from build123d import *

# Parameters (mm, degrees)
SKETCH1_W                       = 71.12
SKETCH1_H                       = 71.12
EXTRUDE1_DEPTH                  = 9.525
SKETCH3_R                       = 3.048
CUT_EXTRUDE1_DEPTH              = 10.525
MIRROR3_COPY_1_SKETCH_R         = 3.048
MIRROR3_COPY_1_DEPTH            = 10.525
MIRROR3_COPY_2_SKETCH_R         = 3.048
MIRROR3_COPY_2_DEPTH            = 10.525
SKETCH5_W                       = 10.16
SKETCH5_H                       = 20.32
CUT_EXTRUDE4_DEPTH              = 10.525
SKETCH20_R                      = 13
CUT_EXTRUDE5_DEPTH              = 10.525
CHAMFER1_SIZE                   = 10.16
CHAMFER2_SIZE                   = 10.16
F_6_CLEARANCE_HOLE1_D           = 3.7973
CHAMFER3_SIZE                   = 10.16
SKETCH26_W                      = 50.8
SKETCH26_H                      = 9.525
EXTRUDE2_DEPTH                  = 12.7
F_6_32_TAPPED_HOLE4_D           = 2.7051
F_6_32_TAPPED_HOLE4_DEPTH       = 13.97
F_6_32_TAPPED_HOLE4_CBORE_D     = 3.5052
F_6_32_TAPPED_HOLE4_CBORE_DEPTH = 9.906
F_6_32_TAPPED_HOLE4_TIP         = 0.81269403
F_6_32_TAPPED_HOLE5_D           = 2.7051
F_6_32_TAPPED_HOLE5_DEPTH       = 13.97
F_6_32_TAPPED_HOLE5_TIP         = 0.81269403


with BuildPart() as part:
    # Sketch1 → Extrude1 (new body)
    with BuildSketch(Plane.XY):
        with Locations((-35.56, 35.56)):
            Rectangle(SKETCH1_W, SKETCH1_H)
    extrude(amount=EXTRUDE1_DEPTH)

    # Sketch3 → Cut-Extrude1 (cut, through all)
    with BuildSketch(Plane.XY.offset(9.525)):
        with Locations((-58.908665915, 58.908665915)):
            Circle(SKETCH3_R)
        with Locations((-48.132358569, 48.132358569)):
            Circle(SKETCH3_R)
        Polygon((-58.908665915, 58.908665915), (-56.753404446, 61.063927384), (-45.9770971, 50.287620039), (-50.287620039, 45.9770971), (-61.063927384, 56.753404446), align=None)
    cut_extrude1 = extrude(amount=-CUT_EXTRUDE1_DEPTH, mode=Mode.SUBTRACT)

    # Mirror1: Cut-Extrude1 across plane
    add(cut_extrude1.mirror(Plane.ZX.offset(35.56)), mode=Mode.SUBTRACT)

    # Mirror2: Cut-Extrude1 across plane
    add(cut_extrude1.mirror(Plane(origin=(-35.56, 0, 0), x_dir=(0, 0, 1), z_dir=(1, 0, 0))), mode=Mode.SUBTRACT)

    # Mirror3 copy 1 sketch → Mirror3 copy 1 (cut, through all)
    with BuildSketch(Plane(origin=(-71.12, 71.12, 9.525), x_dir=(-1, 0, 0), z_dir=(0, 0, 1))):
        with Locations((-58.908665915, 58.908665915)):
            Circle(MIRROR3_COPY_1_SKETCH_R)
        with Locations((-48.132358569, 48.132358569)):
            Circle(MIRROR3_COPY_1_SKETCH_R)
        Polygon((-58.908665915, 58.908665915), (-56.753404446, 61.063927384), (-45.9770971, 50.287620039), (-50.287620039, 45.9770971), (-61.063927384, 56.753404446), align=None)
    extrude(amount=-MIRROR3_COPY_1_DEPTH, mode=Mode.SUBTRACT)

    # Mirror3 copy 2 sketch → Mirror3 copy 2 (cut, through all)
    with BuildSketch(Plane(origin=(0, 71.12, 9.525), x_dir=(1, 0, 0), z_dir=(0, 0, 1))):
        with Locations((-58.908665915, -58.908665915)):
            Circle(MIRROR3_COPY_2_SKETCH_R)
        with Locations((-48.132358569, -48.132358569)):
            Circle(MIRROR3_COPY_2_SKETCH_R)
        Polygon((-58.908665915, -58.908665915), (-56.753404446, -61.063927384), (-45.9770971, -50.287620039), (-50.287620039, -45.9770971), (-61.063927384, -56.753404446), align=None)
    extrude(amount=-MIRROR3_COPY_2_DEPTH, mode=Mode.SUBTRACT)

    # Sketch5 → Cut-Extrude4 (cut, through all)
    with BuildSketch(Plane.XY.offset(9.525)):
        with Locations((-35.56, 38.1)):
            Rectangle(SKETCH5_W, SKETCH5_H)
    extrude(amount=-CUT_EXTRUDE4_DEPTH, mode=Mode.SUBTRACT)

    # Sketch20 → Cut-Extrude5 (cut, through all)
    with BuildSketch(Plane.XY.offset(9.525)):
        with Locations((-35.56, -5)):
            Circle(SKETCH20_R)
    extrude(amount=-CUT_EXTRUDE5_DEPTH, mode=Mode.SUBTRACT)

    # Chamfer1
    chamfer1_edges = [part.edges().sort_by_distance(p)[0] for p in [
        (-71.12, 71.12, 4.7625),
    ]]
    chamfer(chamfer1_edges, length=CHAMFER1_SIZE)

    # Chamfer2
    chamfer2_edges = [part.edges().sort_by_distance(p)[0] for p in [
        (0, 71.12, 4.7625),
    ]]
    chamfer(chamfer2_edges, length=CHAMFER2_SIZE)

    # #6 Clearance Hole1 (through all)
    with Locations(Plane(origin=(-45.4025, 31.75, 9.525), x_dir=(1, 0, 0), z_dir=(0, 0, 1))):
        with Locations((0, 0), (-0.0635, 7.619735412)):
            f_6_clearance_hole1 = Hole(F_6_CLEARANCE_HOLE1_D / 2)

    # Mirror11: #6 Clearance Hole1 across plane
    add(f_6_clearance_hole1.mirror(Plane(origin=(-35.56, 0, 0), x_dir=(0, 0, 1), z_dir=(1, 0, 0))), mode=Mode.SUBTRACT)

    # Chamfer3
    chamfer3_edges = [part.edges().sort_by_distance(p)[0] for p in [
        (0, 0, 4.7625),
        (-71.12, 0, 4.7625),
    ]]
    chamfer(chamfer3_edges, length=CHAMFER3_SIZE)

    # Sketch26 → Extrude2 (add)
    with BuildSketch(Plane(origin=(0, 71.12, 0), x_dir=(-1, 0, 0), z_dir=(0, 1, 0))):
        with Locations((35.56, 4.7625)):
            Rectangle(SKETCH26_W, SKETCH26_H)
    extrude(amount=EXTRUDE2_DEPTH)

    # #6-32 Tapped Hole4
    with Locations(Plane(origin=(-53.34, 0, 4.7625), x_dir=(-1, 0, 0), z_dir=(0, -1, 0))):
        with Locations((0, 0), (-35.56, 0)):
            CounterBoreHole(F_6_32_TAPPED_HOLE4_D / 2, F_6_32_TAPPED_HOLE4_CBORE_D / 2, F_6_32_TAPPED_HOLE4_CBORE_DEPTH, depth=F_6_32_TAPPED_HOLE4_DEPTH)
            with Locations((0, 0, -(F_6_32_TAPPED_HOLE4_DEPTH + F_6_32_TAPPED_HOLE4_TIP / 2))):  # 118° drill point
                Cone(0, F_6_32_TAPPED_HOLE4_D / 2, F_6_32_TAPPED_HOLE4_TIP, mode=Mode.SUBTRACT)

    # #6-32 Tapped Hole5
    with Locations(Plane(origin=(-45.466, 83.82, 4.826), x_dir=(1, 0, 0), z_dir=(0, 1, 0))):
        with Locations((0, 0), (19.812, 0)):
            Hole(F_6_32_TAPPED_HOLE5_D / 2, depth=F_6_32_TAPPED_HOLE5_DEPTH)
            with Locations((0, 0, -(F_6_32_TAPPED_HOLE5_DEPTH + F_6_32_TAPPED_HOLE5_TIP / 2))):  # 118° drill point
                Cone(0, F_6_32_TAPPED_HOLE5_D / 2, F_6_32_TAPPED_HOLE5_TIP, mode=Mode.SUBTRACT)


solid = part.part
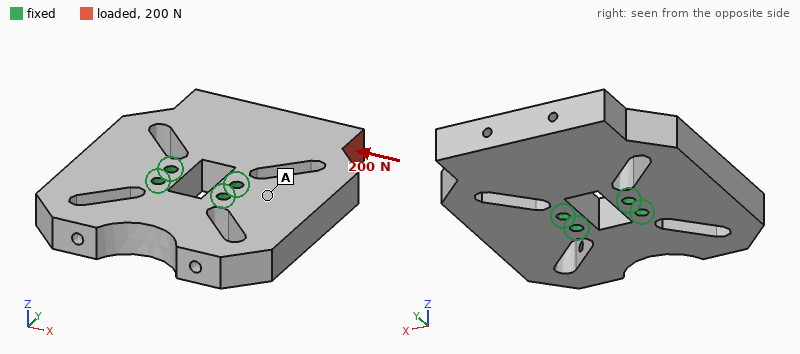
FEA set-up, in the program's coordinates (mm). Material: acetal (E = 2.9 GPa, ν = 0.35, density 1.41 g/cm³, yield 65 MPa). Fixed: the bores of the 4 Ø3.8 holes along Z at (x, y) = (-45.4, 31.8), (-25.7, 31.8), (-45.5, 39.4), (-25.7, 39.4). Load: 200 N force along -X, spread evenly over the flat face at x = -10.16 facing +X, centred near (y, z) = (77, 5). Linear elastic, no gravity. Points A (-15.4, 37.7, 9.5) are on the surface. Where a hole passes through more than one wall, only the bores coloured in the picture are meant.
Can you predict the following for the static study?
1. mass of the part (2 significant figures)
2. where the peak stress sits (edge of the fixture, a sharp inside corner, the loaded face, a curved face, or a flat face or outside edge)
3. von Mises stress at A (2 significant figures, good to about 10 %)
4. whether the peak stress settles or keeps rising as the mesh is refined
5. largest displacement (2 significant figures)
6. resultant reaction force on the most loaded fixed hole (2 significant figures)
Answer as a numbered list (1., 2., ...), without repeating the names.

1. 61 g
2. edge of the fixture
3. 1.0 MPa
4. keeps rising
5. 89 µm
6. 260 N
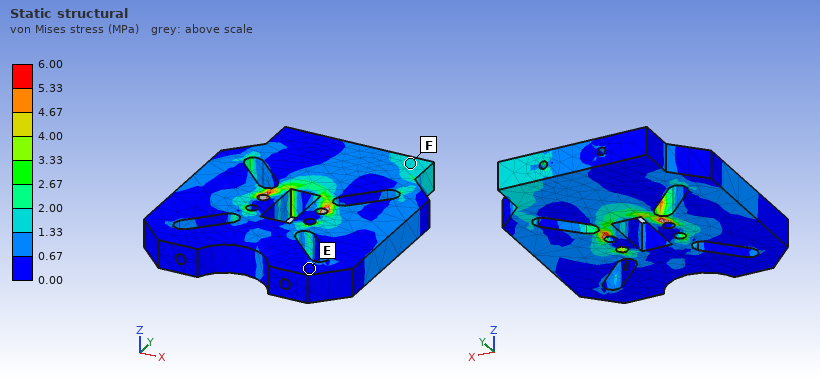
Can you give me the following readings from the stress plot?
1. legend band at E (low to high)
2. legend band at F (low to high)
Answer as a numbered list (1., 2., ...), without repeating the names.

1. 0.00 to 0.67 MPa
2. 1.33 to 2.00 MPa
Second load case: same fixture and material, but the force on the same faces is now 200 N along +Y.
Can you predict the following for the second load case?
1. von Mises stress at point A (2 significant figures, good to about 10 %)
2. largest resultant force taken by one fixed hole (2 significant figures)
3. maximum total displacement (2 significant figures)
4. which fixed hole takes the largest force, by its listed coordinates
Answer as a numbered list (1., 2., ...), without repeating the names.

1. 1.1 MPa
2. 200 N
3. 75 µm
4. (-25.7, 39.4)
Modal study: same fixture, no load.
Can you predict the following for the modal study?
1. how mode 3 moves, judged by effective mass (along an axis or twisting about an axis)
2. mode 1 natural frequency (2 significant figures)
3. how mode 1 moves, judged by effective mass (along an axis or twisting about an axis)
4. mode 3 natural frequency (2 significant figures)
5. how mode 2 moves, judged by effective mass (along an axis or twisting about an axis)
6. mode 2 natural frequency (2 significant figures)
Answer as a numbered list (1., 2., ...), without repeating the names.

1. along Z
2. 820 Hz
3. along Z
4. 1700 Hz
5. twisting about Y
6. 1600 Hz
